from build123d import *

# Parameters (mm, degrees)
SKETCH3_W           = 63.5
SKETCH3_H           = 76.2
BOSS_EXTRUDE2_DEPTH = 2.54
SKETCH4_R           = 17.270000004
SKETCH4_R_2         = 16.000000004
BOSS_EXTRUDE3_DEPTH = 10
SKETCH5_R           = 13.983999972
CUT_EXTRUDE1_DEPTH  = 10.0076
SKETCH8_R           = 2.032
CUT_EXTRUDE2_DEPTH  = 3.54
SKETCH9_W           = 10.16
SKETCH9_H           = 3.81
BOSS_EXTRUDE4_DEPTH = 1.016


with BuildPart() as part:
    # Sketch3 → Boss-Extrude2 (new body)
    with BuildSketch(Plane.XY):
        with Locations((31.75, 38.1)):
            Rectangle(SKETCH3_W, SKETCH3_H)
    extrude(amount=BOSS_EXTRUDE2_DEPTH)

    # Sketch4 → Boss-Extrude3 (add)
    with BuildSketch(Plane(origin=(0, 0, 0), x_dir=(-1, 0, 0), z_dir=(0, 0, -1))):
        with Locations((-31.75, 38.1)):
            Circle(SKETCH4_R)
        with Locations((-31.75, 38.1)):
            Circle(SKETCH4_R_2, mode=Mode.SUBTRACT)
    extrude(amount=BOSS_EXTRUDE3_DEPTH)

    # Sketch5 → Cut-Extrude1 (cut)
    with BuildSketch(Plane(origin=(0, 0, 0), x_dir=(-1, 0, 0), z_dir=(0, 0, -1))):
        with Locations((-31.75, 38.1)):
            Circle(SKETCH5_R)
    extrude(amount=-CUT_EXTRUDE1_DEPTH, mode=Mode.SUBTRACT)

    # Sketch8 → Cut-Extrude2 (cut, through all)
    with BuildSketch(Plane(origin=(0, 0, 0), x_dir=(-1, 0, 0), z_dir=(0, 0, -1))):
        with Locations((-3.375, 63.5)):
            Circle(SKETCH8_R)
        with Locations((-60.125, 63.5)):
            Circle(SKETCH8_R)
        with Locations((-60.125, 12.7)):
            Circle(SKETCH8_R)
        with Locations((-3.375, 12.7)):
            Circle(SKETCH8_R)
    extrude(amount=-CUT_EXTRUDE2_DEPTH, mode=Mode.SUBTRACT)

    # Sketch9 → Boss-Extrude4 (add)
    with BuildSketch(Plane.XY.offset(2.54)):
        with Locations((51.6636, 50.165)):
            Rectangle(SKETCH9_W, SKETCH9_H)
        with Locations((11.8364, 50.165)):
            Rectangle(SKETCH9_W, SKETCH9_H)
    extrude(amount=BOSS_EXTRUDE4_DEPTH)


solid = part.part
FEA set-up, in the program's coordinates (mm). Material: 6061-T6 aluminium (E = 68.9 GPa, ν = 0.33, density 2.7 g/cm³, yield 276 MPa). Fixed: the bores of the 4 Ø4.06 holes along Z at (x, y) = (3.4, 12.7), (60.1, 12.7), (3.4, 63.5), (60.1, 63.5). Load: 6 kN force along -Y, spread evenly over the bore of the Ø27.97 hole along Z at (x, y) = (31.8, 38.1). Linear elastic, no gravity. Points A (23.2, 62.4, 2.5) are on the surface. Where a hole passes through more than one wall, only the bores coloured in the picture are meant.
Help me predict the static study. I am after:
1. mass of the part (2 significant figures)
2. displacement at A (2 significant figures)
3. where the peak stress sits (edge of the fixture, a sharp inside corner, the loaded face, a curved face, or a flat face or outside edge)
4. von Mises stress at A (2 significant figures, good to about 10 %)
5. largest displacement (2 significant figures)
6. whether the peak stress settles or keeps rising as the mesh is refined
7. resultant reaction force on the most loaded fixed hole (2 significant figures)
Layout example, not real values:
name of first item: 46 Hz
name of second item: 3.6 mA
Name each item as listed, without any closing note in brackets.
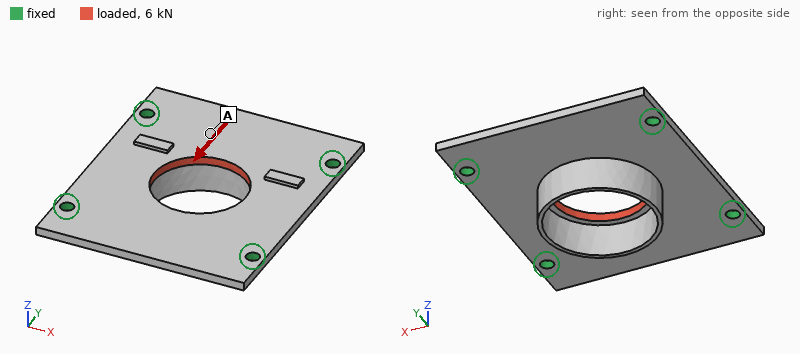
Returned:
mass of the part: 32 g
displacement at A: 19 µm
where the peak stress sits: edge of the fixture
von Mises stress at A: 20 MPa
largest displacement: 24 µm
whether the peak stress settles or keeps rising as the mesh is refined: keeps rising
resultant reaction force on the most loaded fixed hole: 1.5 kN
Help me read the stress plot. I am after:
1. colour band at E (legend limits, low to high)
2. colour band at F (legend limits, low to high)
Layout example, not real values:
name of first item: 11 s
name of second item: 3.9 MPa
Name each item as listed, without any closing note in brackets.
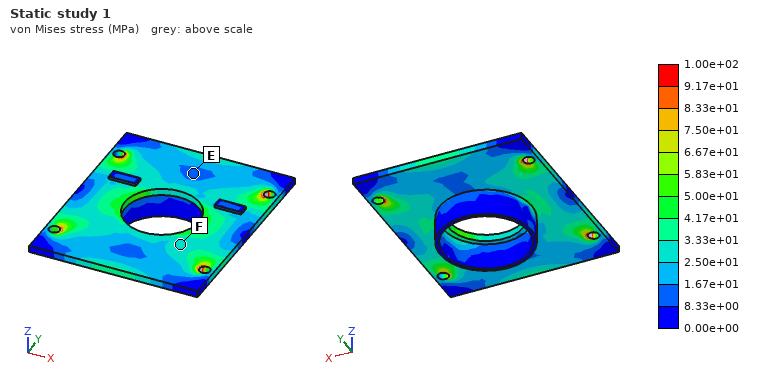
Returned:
colour band at E: 8.33e+00 to 1.67e+01 MPa
colour band at F: 2.50e+01 to 3.33e+01 MPa
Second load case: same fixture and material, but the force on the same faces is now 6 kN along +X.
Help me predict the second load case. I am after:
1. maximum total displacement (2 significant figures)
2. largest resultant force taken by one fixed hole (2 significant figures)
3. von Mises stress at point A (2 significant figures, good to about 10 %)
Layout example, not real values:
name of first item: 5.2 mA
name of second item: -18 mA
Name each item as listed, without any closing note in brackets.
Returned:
maximum total displacement: 24 µm
largest resultant force taken by one fixed hole: 1.6 kN
von Mises stress at point A: 22 MPa
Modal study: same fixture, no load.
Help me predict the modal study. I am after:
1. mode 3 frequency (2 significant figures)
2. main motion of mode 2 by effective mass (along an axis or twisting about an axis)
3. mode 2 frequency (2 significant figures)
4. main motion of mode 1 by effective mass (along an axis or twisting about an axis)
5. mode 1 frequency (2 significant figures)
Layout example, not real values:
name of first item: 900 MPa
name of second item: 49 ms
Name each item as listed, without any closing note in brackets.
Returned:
mode 3 frequency: 4800 Hz
main motion of mode 2 by effective mass: twisting about X
mode 2 frequency: 4200 Hz
main motion of mode 1 by effective mass: along Z
mode 1 frequency: 3600 Hz
